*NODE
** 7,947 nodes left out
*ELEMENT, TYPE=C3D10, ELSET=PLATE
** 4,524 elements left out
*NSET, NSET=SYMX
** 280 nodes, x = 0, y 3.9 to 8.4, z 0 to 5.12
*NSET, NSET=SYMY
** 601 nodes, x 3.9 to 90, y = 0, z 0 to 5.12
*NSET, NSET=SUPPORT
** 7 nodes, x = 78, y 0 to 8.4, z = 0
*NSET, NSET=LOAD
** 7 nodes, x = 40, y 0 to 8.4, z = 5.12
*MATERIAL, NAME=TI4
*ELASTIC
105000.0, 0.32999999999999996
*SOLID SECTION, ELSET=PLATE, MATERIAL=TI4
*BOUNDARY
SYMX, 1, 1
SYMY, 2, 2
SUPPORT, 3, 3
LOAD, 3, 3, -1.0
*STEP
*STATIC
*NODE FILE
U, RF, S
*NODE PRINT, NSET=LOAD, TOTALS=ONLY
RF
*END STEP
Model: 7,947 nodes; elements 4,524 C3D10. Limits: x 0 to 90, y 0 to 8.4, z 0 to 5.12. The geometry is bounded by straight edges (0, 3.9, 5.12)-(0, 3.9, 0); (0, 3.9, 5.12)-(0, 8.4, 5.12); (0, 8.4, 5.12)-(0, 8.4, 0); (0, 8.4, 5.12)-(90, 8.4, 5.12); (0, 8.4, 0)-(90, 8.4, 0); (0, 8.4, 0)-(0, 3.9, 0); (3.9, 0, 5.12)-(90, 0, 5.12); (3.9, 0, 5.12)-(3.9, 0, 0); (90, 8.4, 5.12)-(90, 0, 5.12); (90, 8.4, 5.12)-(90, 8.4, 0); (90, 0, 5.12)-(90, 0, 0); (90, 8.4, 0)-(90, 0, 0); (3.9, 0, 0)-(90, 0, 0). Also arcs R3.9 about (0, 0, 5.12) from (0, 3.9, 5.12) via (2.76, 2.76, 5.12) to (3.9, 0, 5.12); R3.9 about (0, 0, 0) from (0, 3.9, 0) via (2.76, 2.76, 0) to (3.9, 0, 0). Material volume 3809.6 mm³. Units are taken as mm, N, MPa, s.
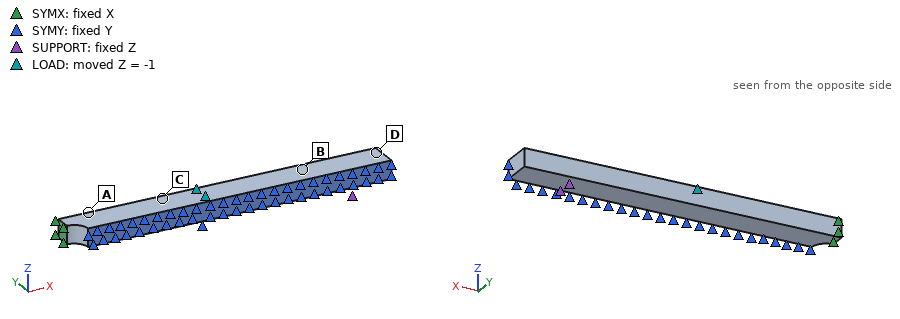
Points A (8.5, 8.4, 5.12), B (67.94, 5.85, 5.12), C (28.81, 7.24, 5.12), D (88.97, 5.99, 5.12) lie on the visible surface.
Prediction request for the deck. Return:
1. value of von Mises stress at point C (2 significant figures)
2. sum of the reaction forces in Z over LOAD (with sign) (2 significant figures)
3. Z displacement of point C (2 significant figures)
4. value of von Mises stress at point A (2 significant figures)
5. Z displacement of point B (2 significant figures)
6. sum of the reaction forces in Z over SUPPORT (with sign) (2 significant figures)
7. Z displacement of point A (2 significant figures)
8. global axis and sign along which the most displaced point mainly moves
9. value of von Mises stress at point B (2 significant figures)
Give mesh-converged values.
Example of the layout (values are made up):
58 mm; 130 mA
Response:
130 MPa; -120 N; -1.2 mm; 140 MPa; -0.29 mm; 120 N; -1.4 mm; -Z; 33 MPa
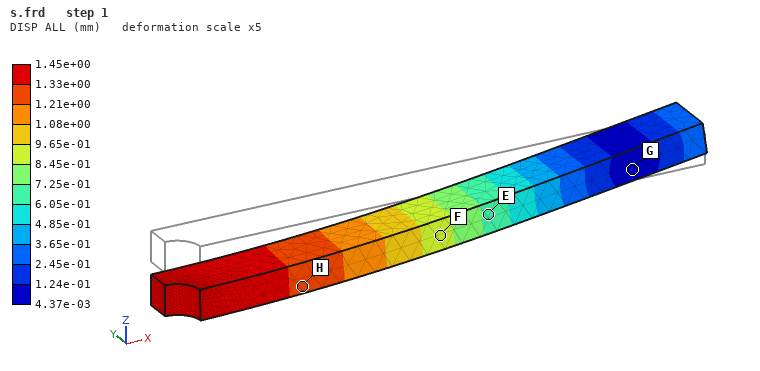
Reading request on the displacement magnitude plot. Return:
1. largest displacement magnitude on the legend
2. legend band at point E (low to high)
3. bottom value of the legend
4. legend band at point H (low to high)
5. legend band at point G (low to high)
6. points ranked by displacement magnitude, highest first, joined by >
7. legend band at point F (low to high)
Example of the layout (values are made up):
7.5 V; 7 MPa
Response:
1.45e+00 mm; 6.05e-01 to 7.25e-01 mm; 4.37e-03 mm; 1.21e+00 to 1.33e+00 mm; 4.37e-03 to 1.24e-01 mm; H > F > E > G; 8.45e-01 to 9.65e-01 mm
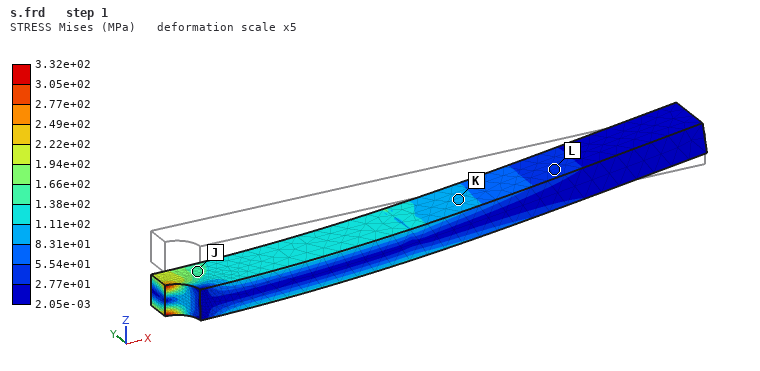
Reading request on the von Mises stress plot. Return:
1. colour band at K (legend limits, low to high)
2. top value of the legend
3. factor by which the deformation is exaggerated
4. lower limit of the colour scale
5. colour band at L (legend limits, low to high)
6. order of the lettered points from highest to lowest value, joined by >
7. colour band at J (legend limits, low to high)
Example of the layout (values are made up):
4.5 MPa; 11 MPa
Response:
8.31e+01 to 1.11e+02 MPa; 3.32e+02 MPa; 5; 2.05e-03 MPa; 2.77e+01 to 5.54e+01 MPa; J > K > L; 1.38e+02 to 1.66e+02 MPa
